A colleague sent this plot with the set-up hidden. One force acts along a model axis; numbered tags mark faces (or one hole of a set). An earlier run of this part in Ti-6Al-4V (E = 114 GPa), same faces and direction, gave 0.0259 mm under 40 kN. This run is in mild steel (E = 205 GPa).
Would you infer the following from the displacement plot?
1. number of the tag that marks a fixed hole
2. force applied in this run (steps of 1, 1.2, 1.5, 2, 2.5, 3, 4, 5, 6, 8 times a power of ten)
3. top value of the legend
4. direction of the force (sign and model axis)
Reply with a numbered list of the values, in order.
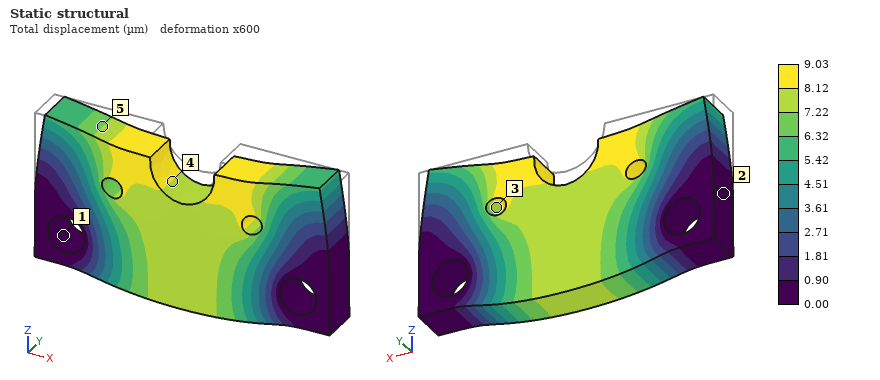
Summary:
1. 1
2. 25 kN
3. 9.03 µm
4. -Z
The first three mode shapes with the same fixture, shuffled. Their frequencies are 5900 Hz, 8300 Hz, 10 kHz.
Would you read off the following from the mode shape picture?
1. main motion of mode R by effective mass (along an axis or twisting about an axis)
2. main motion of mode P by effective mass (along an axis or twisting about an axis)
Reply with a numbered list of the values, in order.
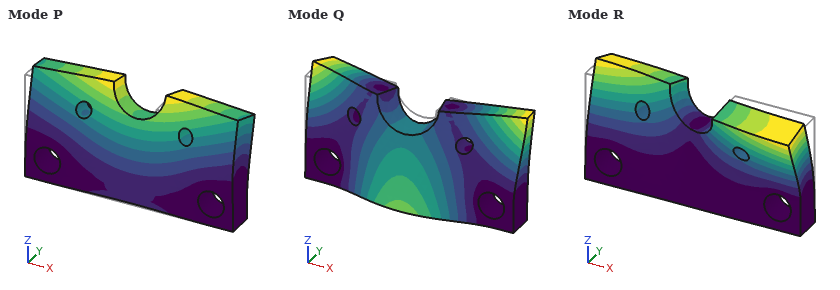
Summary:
1. twisting about Z
2. along Y
